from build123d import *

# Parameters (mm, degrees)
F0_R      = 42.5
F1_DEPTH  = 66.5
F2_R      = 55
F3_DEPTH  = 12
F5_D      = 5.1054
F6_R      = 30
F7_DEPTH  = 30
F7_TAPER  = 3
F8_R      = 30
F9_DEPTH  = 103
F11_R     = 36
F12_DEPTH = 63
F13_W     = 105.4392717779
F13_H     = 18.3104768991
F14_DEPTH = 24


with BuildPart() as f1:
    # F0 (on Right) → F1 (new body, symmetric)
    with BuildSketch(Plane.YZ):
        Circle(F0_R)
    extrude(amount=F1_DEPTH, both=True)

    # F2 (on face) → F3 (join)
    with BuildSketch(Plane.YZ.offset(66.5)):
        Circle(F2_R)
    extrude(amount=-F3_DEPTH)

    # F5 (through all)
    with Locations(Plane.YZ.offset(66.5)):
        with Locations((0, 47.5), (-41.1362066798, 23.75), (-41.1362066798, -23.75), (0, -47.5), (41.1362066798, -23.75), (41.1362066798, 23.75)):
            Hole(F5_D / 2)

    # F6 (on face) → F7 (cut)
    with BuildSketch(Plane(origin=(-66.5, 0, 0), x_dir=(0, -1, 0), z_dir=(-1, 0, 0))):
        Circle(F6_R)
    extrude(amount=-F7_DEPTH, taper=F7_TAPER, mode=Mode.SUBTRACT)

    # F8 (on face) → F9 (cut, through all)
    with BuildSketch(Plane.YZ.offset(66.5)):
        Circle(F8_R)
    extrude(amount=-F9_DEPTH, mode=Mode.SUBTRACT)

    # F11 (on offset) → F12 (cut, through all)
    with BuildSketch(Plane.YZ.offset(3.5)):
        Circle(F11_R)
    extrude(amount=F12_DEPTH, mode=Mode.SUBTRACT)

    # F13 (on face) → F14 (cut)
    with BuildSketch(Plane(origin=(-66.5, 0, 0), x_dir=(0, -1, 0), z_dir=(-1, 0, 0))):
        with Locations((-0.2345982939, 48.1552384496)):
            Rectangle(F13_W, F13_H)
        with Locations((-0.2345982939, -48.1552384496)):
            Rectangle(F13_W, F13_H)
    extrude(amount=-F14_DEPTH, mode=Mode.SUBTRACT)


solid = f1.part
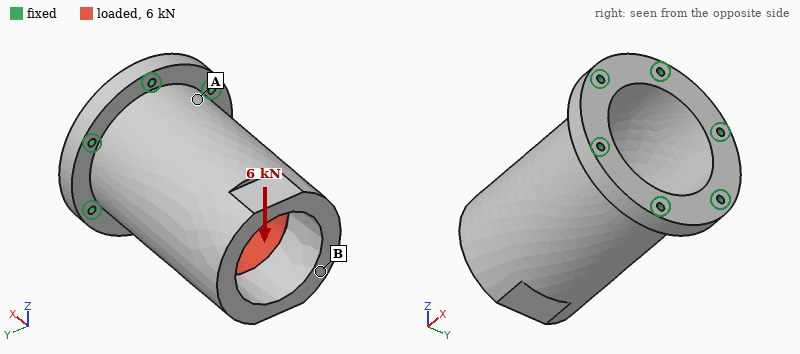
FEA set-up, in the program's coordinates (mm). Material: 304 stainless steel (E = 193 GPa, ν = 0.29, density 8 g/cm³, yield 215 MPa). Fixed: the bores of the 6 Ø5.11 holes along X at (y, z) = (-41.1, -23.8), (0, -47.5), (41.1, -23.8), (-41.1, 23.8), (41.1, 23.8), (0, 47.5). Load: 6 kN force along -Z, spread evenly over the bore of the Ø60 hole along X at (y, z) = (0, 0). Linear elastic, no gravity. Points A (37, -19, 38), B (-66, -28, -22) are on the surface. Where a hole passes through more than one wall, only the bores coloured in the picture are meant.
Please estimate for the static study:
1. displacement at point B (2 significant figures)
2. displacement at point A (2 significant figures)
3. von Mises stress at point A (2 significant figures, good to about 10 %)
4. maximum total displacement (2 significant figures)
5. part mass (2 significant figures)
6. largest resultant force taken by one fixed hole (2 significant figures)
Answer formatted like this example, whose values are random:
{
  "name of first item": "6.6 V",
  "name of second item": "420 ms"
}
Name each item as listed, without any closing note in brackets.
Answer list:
{
  "displacement at point B": "20 µm",
  "displacement at point A": "4.9 µm",
  "von Mises stress at point A": "9.2 MPa",
  "maximum total displacement": "20 µm",
  "part mass": "2.8 kg",
  "largest resultant force taken by one fixed hole": "3.6 kN"
}
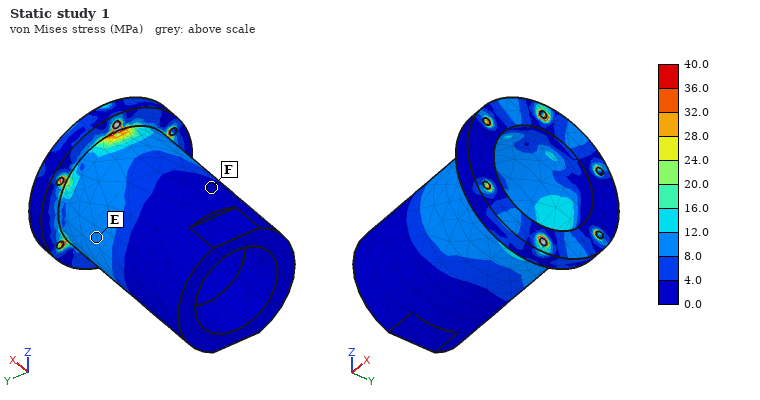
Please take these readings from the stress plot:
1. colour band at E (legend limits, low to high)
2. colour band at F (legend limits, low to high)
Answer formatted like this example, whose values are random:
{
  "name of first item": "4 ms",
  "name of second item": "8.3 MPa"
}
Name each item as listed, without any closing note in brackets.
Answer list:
{
  "colour band at E": "8.0 to 12.0 MPa",
  "colour band at F": "0.0 to 4.0 MPa"
}
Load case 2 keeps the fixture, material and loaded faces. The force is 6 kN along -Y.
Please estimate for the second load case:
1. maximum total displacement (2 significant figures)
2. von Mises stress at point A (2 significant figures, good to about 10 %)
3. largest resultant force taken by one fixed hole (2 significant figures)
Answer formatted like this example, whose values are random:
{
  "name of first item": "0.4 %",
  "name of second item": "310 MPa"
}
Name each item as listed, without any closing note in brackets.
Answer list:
{
  "maximum total displacement": "20 µm",
  "von Mises stress at point A": "10 MPa",
  "largest resultant force taken by one fixed hole": "3.1 kN"
}
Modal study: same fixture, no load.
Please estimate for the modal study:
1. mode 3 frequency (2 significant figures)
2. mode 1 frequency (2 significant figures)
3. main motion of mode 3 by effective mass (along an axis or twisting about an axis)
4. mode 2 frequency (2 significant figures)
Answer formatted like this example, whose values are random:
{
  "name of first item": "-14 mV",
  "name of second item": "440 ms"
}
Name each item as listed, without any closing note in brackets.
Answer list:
{
  "mode 3 frequency": "5200 Hz",
  "mode 1 frequency": "2100 Hz",
  "main motion of mode 3 by effective mass": "twisting about X",
  "mode 2 frequency": "2100 Hz"
}
